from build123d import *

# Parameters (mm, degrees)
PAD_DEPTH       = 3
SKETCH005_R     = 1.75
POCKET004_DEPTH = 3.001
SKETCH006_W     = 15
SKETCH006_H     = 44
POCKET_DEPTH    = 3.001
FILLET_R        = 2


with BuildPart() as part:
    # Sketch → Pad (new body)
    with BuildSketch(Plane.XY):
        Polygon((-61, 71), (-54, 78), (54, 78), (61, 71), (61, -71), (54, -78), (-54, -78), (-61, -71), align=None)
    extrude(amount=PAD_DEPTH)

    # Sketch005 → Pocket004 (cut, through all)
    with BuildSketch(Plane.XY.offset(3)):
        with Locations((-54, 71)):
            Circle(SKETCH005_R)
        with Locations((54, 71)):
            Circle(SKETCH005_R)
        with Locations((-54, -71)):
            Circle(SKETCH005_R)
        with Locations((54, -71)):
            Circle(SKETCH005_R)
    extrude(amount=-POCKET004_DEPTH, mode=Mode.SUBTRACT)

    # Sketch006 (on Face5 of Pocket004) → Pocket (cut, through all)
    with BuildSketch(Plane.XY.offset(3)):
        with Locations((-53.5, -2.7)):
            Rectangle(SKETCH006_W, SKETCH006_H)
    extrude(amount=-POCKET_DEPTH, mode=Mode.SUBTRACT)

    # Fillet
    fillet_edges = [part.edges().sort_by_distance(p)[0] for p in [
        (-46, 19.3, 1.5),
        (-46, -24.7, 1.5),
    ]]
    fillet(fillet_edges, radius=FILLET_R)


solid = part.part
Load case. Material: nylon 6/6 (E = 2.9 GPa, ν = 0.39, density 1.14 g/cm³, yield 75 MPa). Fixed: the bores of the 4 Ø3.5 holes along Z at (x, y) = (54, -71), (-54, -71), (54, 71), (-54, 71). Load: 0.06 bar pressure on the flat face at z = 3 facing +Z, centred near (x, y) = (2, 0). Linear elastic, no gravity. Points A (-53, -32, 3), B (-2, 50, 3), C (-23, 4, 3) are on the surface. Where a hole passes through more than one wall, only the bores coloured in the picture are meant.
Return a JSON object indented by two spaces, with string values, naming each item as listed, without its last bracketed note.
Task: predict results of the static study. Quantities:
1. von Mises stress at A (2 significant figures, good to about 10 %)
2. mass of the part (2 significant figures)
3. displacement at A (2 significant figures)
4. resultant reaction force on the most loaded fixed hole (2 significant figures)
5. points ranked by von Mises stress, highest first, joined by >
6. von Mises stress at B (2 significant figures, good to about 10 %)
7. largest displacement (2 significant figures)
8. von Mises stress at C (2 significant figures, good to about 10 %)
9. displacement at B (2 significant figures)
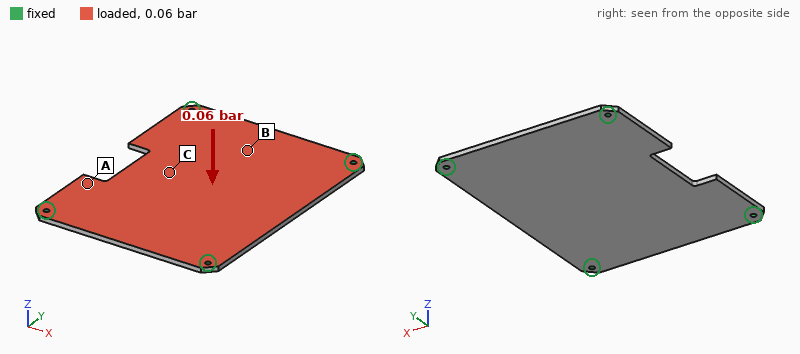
{
  "von Mises stress at A": "1.3 MPa",
  "mass of the part": "62 g",
  "displacement at A": "1.1 mm",
  "resultant reaction force on the most loaded fixed hole": "28 N",
  "points ranked by von Mises stress, highest first, joined by >": "C > B > A",
  "von Mises stress at B": "2.8 MPa",
  "largest displacement": "1.9 mm",
  "von Mises stress at C": "4.3 MPa",
  "displacement at B": "1.1 mm"
}
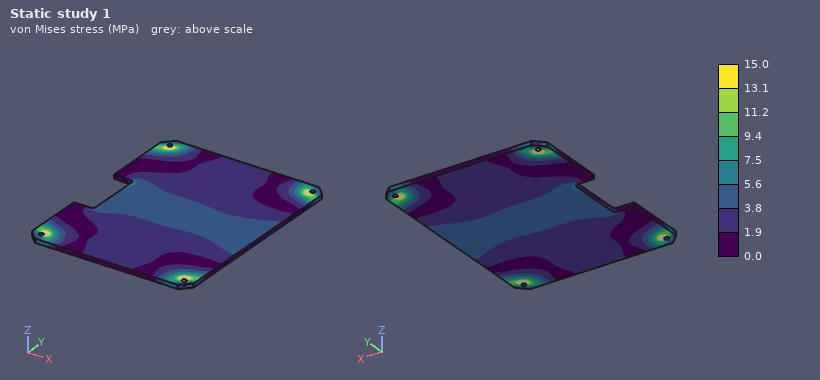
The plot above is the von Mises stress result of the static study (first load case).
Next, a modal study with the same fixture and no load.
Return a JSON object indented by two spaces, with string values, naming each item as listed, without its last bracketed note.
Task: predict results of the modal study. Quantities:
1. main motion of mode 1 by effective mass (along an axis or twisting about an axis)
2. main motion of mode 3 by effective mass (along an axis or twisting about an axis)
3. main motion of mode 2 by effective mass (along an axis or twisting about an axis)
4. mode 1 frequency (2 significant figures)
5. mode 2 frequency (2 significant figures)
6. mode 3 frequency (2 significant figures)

{
  "main motion of mode 1 by effective mass": "along Z",
  "main motion of mode 3 by effective mass": "twisting about X",
  "main motion of mode 2 by effective mass": "twisting about Y",
  "mode 1 frequency": "180 Hz",
  "mode 2 frequency": "310 Hz",
  "mode 3 frequency": "390 Hz"
}
